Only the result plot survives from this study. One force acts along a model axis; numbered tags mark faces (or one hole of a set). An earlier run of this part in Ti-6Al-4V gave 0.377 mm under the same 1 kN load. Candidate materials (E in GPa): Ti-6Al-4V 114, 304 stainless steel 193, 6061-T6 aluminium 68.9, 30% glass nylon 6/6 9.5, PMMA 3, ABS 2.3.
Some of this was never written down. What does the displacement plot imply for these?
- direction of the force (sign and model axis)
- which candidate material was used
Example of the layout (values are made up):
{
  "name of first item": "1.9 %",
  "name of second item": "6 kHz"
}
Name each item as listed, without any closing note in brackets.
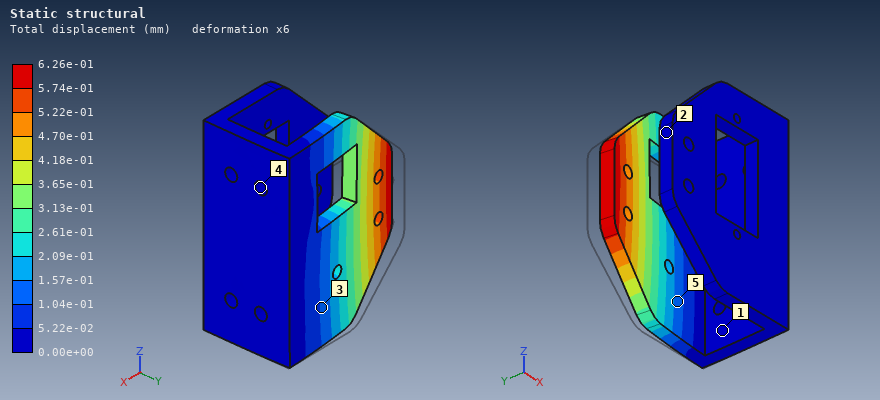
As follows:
{
  "direction of the force": "-Y",
  "which candidate material was used": "6061-T6 aluminium"
}
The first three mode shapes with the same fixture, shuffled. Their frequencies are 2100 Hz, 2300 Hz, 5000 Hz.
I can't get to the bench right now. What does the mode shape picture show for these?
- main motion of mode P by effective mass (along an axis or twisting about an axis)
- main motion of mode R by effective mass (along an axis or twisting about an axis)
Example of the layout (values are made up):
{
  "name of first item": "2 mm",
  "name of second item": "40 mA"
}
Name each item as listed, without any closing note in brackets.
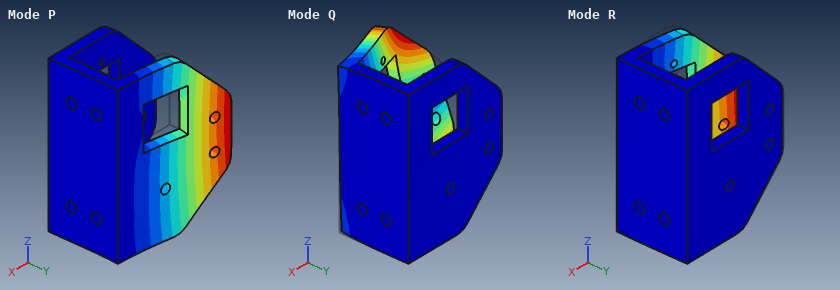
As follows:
{
  "main motion of mode P by effective mass": "along Y",
  "main motion of mode R by effective mass": "along Y"
}
